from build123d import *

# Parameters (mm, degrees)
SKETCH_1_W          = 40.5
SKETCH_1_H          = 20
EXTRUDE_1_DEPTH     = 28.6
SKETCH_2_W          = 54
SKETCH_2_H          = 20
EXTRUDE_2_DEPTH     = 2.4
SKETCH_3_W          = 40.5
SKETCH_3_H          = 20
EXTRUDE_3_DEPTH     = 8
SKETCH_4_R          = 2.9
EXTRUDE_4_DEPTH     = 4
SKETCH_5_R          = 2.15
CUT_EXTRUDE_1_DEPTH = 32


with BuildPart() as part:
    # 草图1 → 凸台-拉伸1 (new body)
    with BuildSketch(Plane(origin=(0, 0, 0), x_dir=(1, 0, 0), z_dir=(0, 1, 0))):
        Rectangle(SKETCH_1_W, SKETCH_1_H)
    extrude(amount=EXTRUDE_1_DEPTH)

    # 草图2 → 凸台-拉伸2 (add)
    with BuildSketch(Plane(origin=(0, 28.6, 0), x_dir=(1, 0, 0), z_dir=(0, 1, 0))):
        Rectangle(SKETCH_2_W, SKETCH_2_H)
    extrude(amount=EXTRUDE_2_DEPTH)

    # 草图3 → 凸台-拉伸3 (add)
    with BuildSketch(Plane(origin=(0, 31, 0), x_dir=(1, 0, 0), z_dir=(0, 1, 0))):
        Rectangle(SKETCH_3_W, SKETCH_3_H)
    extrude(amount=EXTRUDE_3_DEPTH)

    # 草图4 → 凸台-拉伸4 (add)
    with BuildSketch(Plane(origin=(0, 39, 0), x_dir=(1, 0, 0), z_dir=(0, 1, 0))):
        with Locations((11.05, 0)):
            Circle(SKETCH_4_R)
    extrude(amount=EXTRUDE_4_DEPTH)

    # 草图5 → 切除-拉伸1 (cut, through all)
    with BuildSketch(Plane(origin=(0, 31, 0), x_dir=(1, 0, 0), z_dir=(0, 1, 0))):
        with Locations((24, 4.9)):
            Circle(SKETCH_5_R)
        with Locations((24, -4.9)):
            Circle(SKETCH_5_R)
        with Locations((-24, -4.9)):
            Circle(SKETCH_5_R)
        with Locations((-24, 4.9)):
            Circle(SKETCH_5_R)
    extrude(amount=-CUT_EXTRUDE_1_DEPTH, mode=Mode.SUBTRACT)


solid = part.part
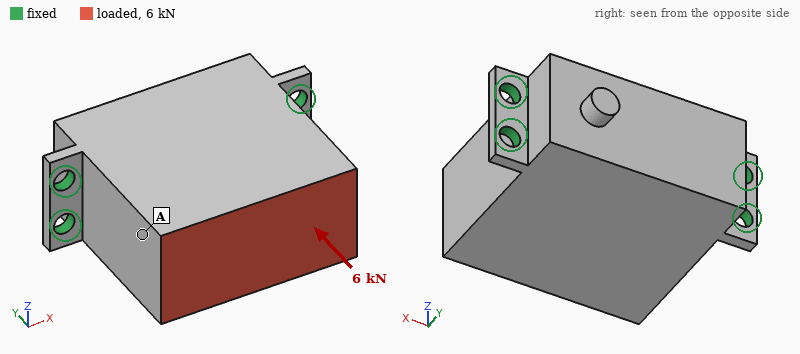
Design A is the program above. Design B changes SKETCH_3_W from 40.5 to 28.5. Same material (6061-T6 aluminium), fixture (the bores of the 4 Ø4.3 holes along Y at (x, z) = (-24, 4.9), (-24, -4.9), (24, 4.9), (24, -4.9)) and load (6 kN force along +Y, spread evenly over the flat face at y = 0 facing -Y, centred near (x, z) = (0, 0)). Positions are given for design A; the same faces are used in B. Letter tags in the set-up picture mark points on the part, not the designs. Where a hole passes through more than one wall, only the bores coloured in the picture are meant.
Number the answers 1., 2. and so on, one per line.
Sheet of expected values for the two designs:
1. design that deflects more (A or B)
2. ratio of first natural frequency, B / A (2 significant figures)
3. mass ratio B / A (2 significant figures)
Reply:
1. B
2. 0.91
3. 0.94
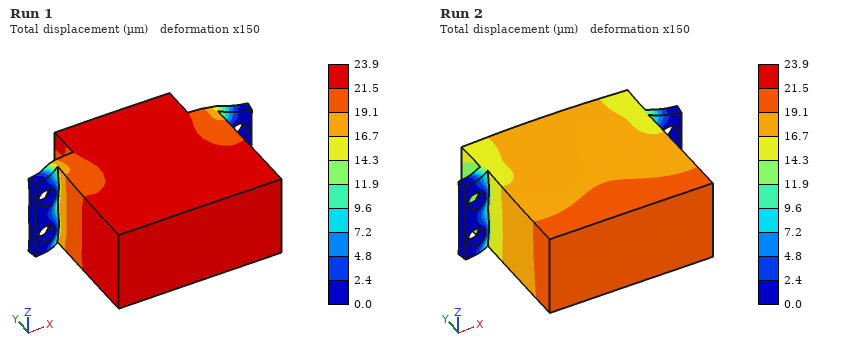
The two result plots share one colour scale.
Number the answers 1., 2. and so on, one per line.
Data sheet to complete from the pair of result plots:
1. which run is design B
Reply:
1. Run 1
